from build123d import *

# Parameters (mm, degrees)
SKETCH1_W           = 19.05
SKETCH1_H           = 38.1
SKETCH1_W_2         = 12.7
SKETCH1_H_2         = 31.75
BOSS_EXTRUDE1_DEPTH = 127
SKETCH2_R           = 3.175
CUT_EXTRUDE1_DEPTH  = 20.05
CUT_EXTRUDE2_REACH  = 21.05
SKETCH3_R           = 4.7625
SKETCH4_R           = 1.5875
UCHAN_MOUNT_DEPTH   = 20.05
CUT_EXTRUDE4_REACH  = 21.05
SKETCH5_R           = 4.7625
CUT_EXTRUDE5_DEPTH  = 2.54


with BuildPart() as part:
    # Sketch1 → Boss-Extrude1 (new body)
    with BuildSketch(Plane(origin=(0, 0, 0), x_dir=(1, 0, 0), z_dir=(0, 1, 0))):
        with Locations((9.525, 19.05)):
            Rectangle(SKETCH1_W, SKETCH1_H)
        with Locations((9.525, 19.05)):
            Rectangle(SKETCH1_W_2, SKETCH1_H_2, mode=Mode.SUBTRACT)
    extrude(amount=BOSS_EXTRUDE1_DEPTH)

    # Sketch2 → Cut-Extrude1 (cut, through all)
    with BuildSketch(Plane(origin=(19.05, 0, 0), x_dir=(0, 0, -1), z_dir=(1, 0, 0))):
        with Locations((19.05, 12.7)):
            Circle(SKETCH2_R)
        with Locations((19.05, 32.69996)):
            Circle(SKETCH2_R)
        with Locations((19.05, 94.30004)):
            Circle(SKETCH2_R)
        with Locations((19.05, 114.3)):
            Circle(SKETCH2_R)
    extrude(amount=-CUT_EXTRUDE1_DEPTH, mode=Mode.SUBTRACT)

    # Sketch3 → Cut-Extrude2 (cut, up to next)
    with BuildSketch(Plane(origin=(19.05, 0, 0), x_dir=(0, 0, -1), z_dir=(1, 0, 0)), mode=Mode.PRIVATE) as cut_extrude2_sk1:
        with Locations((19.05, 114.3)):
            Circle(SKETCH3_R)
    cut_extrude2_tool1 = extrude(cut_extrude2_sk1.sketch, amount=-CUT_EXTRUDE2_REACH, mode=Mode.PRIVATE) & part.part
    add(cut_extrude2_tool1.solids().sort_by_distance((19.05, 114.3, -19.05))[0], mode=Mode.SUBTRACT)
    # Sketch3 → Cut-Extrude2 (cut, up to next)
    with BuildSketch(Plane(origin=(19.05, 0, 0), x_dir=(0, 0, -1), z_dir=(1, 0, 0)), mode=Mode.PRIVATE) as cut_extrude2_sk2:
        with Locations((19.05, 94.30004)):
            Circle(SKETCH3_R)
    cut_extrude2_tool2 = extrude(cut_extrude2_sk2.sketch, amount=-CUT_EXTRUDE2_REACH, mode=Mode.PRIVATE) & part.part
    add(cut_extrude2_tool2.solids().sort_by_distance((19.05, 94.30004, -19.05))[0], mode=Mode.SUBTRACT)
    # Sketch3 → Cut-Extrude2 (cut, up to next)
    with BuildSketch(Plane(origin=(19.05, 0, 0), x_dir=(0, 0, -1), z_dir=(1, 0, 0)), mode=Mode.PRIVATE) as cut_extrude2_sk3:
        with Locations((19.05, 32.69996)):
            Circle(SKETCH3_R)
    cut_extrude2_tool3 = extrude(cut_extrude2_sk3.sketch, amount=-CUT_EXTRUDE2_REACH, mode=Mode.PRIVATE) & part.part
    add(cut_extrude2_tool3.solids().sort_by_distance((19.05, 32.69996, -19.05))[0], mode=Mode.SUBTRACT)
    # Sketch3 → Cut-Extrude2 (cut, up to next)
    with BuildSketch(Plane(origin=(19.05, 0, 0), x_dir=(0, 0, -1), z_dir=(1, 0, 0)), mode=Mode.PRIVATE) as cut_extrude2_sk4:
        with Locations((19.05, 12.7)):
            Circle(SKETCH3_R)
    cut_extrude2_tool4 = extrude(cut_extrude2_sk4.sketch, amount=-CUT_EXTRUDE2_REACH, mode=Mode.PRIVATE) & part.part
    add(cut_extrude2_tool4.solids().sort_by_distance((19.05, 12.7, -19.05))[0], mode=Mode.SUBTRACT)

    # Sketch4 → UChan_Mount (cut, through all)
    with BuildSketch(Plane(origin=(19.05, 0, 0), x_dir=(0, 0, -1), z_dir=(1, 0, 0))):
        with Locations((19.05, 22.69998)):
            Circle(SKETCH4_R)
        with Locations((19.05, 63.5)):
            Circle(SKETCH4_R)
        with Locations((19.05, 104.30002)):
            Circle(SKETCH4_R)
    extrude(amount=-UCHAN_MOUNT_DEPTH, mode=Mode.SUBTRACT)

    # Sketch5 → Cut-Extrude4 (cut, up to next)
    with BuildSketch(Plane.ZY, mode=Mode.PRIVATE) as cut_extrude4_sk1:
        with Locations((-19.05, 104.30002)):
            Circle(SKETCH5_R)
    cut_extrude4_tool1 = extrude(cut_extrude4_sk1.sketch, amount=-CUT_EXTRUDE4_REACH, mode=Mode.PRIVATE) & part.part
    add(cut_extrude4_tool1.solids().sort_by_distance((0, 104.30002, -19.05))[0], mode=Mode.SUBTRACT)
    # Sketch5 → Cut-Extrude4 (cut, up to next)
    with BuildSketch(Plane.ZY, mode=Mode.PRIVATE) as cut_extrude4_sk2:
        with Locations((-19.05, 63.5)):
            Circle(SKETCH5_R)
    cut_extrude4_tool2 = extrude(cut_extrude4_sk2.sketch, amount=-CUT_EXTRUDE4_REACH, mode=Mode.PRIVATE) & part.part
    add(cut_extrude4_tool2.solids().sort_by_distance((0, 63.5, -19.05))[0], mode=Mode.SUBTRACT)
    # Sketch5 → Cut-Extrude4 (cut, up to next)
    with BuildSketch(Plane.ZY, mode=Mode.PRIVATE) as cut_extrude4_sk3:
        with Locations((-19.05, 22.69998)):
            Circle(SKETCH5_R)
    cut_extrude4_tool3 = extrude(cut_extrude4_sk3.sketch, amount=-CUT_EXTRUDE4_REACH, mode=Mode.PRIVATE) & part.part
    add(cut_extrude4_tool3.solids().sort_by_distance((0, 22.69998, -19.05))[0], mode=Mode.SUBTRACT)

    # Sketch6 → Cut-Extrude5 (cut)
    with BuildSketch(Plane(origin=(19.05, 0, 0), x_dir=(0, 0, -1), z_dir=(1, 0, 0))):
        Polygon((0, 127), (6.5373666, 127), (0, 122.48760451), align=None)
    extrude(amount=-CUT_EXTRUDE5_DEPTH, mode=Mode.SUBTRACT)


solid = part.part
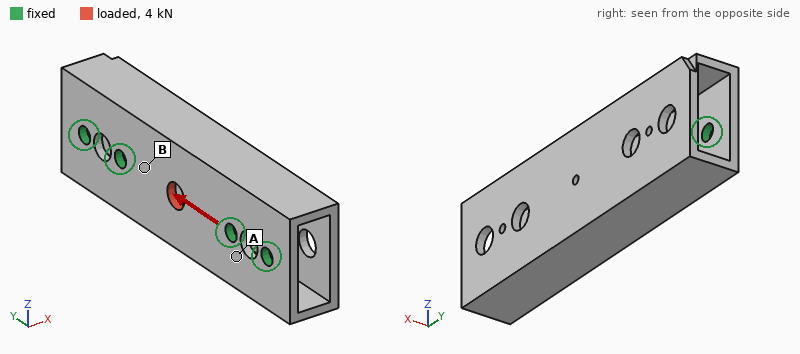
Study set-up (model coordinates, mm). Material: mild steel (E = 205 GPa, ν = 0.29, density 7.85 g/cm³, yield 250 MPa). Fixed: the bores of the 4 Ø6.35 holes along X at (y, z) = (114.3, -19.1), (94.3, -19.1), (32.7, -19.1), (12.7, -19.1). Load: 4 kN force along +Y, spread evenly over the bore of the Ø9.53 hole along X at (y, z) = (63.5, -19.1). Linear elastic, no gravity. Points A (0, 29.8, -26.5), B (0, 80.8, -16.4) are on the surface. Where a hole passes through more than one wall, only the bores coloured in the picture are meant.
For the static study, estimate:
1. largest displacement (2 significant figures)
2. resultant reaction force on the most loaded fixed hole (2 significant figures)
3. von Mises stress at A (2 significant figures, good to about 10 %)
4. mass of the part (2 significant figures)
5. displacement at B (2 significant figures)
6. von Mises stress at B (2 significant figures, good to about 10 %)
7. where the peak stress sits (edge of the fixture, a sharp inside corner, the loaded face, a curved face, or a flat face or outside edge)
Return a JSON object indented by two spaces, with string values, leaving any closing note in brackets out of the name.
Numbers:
{
  "largest displacement": "4.1 µm",
  "resultant reaction force on the most loaded fixed hole": "1.5 kN",
  "von Mises stress at A": "11 MPa",
  "mass of the part": "310 g",
  "displacement at B": "1.7 µm",
  "von Mises stress at B": "31 MPa",
  "where the peak stress sits": "the loaded face"
}
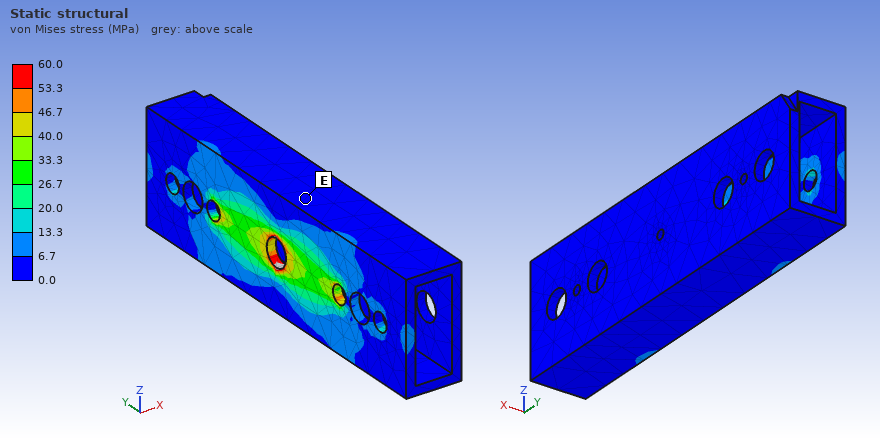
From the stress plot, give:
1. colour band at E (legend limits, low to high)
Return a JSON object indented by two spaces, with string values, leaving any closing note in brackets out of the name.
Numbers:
{
  "colour band at E": "0.0 to 6.7 MPa"
}
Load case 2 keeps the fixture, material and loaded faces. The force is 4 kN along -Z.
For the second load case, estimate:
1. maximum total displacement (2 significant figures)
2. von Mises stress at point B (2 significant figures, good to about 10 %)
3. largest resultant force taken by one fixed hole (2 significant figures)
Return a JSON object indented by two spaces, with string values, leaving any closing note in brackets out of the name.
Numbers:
{
  "maximum total displacement": "9.5 µm",
  "von Mises stress at point B": "25 MPa",
  "largest resultant force taken by one fixed hole": "2.2 kN"
}
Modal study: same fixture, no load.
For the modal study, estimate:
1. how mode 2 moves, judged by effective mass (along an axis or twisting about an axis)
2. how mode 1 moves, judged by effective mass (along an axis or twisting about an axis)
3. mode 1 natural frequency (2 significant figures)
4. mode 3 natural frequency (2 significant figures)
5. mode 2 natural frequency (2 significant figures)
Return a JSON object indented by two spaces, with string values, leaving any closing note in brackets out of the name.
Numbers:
{
  "how mode 2 moves, judged by effective mass": "along X",
  "how mode 1 moves, judged by effective mass": "along Z",
  "mode 1 natural frequency": "2200 Hz",
  "mode 3 natural frequency": "4500 Hz",
  "mode 2 natural frequency": "4100 Hz"
}
